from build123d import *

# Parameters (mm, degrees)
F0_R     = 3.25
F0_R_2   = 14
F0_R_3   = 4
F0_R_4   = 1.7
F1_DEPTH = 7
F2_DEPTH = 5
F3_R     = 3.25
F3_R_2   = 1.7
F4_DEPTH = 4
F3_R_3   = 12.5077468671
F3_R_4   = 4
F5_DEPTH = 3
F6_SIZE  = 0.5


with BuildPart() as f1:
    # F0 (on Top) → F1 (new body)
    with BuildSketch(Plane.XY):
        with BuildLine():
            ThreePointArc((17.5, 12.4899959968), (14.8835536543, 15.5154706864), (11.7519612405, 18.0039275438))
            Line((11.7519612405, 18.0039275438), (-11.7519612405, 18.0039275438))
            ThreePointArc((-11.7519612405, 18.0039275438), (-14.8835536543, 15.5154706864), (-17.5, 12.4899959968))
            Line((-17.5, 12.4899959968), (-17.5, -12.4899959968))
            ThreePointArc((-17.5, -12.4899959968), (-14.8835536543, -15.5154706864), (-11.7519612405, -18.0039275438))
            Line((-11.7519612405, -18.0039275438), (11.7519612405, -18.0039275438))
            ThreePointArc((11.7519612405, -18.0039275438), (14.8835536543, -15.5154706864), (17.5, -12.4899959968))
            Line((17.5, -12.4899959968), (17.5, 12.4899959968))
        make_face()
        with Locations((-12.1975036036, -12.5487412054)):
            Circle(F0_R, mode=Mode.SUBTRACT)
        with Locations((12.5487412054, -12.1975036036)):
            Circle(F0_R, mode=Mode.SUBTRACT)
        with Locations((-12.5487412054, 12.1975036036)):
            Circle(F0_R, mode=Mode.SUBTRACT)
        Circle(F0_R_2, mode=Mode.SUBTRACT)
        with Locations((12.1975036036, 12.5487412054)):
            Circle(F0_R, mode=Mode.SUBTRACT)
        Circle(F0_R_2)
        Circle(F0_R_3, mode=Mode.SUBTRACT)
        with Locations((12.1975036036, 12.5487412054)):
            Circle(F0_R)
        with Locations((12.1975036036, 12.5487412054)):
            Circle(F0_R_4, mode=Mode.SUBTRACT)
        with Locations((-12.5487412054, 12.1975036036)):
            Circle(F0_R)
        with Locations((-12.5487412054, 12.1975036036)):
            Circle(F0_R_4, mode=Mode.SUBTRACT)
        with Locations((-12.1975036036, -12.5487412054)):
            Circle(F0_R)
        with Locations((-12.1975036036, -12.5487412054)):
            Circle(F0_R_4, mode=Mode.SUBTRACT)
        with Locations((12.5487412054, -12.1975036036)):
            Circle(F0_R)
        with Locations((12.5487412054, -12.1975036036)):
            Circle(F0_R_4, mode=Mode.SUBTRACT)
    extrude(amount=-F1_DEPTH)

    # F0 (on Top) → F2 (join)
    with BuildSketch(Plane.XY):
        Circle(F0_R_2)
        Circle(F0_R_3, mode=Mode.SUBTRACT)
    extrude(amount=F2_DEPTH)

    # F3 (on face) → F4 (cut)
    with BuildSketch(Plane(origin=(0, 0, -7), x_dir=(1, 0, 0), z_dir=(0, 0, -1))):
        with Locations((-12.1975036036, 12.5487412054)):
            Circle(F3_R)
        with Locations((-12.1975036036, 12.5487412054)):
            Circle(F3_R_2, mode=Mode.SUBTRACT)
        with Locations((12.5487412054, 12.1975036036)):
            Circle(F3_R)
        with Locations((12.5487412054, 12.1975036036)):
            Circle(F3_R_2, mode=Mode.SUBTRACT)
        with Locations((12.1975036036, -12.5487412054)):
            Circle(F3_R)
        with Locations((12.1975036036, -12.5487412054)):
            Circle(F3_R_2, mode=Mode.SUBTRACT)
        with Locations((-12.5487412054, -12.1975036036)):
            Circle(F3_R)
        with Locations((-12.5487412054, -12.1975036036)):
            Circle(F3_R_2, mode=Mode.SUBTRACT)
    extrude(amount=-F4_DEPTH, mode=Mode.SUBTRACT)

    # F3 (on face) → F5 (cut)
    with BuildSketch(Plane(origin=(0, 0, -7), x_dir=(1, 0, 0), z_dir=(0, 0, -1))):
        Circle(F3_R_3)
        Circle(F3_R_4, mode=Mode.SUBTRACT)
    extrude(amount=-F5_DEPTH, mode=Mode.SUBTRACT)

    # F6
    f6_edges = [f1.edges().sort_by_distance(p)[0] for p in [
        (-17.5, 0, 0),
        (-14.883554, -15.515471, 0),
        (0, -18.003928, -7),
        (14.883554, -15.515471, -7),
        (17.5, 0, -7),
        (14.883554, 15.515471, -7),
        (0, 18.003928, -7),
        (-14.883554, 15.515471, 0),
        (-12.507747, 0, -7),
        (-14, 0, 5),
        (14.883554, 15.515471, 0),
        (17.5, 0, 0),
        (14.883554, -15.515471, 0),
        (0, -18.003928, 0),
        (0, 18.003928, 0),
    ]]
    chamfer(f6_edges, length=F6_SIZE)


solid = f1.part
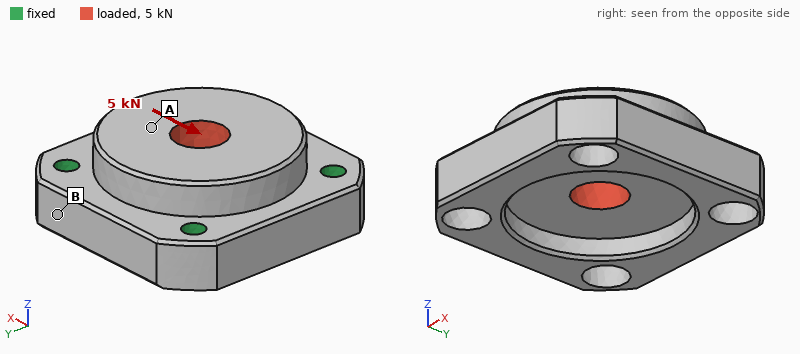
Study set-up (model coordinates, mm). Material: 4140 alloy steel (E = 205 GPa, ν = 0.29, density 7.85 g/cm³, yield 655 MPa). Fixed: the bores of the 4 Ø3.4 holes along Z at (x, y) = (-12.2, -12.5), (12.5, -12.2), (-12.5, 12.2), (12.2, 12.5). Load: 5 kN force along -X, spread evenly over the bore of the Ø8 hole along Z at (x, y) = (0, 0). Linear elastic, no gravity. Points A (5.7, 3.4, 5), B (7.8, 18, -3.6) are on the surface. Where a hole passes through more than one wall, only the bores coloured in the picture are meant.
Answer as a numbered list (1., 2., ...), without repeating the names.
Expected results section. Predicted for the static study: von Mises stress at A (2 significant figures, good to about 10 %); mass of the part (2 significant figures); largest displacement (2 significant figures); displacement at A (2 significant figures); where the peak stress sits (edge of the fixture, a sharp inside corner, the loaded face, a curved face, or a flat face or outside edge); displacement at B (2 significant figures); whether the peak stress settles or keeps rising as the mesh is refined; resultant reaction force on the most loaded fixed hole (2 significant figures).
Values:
1. 19 MPa
2. 70 g
3. 2.8 µm
4. 2.4 µm
5. edge of the fixture
6. 0.57 µm
7. keeps rising
8. 1.3 kN
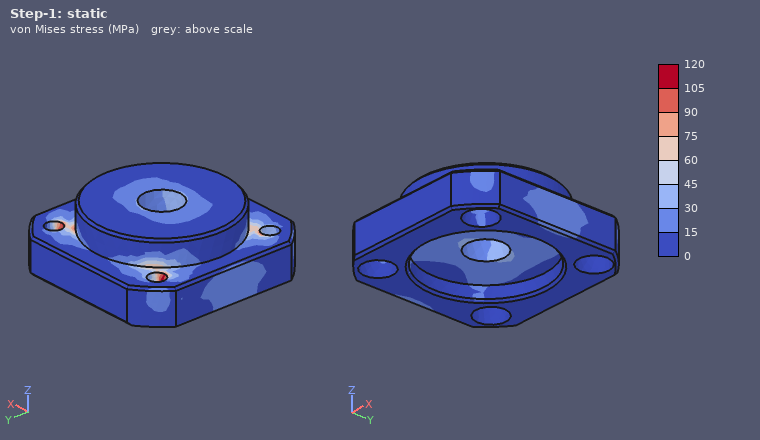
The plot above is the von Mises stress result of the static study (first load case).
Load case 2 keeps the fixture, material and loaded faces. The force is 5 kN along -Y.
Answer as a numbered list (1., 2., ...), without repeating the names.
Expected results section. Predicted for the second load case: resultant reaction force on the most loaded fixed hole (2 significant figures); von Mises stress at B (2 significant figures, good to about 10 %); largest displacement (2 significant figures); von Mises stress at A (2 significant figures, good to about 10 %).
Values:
1. 1.3 kN
2. 14 MPa
3. 2.8 µm
4. 15 MPa
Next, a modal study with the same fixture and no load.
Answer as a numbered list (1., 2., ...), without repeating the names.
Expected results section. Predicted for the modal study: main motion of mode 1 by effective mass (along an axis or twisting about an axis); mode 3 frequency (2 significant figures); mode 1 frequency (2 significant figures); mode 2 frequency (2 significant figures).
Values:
1. along Z
2. 32 kHz
3. 25 kHz
4. 32 kHz
